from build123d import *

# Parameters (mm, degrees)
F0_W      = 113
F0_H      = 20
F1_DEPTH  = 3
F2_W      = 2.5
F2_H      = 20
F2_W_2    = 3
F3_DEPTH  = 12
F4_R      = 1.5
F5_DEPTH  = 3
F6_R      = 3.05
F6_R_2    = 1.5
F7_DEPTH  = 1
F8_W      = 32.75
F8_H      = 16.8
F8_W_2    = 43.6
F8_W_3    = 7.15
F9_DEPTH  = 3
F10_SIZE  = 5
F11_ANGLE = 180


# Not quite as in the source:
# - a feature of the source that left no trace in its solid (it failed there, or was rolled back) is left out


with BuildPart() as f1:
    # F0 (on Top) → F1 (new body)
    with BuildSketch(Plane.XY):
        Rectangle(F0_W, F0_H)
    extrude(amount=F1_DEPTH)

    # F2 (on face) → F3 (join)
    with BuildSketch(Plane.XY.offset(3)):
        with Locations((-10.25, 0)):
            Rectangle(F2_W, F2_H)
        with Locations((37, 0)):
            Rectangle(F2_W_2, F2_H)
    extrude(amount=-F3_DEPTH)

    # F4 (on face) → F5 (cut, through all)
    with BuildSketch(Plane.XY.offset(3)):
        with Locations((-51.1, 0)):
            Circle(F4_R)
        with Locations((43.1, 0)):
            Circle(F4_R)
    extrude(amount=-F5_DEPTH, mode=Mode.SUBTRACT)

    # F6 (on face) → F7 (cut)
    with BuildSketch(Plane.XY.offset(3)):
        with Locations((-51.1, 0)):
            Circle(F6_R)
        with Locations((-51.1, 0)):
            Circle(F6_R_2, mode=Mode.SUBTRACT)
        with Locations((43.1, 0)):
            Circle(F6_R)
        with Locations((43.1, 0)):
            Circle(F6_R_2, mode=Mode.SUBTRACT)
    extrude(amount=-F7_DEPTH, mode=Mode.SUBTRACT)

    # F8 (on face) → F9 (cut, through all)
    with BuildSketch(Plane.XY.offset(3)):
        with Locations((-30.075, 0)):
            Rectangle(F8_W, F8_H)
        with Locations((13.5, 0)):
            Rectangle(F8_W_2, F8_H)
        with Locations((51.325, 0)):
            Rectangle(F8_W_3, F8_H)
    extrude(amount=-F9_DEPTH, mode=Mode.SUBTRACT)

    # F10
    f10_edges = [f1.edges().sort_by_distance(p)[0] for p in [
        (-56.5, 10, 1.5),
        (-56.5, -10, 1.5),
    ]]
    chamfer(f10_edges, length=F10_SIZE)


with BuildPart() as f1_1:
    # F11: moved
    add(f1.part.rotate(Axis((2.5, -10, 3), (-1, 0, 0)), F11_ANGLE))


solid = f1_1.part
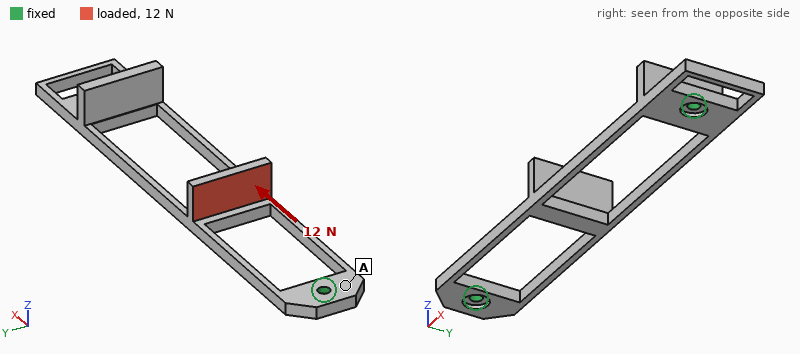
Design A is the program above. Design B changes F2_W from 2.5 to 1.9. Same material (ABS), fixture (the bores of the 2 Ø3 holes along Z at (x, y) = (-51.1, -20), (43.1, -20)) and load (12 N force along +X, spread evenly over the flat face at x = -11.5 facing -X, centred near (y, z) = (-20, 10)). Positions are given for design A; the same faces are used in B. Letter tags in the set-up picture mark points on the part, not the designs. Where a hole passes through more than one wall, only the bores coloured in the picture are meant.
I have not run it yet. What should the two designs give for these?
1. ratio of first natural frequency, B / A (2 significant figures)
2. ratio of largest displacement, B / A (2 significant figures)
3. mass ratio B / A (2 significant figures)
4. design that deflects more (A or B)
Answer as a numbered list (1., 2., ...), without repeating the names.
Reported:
1. 1.1
2. 1.1
3. 0.97
4. B
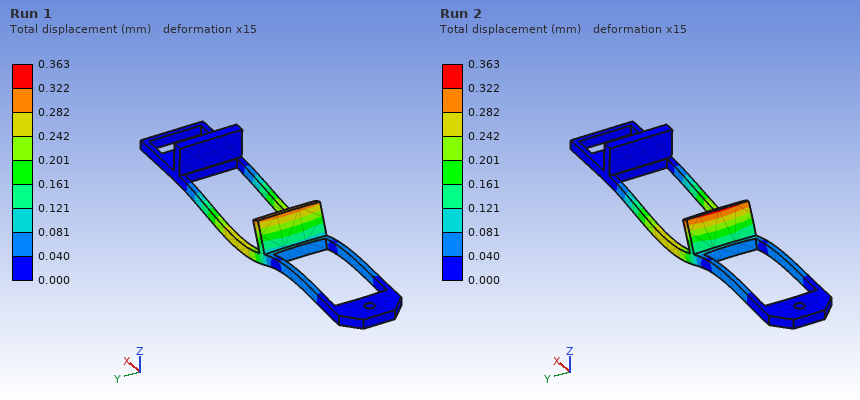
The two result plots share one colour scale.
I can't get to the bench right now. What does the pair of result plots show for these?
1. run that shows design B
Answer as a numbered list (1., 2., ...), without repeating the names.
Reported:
1. Run 2
